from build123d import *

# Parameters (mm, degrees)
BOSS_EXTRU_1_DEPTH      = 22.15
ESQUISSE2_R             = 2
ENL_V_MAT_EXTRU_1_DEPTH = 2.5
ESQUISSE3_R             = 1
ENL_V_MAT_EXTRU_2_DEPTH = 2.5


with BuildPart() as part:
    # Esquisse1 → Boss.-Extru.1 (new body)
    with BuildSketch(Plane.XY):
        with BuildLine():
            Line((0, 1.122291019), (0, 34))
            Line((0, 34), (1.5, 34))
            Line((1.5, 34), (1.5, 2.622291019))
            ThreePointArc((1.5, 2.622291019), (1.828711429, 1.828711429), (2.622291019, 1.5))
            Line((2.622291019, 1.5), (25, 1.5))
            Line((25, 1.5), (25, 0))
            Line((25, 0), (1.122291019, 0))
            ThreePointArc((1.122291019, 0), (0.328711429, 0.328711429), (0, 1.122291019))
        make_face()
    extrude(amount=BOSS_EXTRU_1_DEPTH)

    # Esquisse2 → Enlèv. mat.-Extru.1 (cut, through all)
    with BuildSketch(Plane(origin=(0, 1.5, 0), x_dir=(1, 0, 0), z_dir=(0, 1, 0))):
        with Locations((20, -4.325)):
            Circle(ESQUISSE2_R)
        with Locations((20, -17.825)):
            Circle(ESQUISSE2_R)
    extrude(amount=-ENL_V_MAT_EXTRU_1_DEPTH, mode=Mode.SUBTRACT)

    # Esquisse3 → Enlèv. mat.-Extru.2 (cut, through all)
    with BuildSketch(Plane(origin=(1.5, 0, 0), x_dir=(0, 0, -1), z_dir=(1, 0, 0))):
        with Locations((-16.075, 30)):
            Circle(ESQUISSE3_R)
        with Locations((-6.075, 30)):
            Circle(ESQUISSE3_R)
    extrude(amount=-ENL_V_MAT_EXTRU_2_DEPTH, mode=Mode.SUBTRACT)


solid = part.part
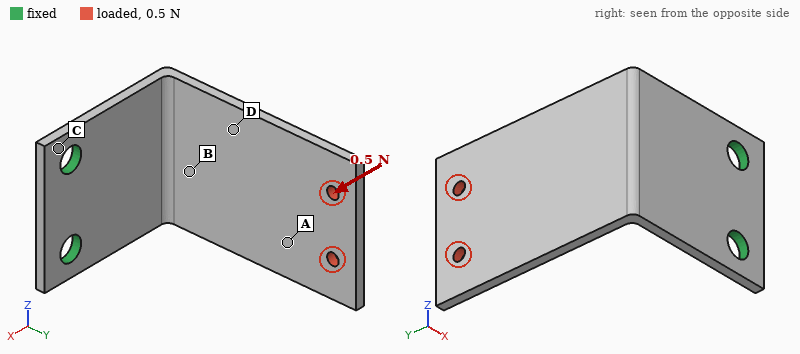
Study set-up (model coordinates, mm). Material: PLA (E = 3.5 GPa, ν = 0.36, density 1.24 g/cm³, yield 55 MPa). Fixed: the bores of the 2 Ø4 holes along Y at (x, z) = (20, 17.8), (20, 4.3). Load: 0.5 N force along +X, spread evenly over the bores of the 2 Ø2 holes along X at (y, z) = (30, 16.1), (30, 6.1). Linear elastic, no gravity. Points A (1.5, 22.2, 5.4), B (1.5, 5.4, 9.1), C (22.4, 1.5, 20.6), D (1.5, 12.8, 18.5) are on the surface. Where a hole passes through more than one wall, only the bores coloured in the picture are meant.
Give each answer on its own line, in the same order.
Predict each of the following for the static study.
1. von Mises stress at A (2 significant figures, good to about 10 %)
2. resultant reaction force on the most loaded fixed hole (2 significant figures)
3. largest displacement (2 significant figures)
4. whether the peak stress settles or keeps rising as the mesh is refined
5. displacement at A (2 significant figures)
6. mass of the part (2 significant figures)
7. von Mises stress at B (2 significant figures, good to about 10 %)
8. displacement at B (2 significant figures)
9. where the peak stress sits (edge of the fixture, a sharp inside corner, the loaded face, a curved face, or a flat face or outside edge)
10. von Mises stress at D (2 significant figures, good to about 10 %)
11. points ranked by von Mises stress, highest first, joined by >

0.48 MPa
0.27 N
0.57 mm
keeps rising
0.34 mm
2.3 g
1.4 MPa
0.11 mm
edge of the fixture
0.99 MPa
B > D > A > C
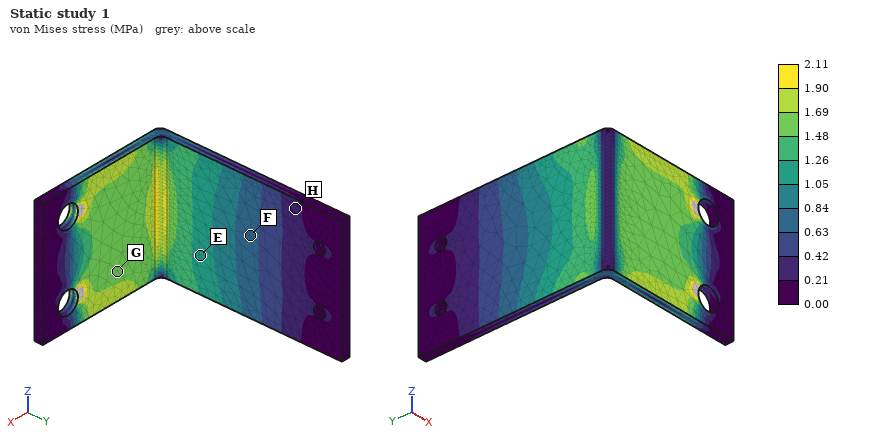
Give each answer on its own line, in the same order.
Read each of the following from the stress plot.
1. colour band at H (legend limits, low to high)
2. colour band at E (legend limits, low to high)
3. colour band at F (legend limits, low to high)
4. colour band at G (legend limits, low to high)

0.21 to 0.42 MPa
1.05 to 1.26 MPa
0.63 to 0.84 MPa
1.48 to 1.69 MPa
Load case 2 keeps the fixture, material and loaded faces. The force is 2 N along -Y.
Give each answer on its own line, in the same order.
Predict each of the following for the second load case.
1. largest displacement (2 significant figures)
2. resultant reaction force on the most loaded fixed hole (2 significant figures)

0.49 mm
1.0 N
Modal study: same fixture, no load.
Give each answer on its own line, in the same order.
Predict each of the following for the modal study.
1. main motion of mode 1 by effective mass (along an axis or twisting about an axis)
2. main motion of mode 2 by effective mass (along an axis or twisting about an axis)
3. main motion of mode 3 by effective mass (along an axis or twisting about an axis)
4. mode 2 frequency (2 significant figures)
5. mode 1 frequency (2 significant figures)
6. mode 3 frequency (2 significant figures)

along X
along Z
along Y
380 Hz
210 Hz
690 Hz
